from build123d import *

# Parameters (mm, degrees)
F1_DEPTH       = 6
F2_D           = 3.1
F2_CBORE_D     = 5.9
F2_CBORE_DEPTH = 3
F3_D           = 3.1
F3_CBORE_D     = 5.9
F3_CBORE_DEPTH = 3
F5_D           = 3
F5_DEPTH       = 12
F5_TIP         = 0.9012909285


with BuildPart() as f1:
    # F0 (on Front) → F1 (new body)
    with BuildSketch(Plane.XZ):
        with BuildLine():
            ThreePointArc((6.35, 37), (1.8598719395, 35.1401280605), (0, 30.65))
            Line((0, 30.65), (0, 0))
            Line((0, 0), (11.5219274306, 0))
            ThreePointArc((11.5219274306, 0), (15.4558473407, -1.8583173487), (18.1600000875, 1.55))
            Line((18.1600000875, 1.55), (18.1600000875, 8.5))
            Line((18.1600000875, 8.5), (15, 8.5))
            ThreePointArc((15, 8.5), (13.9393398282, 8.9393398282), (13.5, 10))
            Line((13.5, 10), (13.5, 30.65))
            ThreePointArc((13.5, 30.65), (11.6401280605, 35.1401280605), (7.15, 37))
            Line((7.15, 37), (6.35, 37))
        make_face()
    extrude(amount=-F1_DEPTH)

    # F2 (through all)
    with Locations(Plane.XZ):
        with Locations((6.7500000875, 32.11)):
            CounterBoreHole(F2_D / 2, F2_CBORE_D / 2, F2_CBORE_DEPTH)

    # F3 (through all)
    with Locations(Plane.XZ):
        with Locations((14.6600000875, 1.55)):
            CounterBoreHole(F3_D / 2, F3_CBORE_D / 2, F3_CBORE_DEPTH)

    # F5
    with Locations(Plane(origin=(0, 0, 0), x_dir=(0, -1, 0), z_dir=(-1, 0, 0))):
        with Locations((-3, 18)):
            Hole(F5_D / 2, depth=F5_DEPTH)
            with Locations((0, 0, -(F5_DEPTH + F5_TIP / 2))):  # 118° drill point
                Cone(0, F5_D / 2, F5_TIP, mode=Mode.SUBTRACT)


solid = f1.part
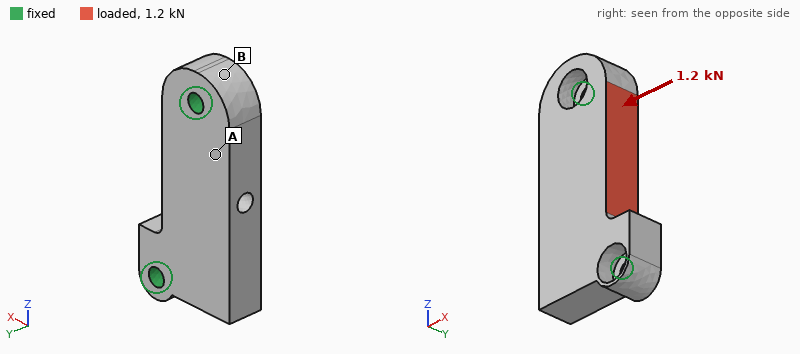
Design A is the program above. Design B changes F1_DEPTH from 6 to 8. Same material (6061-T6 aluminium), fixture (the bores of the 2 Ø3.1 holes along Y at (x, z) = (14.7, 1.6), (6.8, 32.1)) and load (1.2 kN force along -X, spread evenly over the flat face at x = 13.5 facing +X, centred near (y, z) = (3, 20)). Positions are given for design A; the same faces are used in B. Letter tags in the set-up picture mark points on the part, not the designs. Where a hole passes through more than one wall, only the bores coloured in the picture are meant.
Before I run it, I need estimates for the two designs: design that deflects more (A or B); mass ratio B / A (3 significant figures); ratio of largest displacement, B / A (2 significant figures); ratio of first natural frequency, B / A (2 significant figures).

A
1.36
0.53
1.3
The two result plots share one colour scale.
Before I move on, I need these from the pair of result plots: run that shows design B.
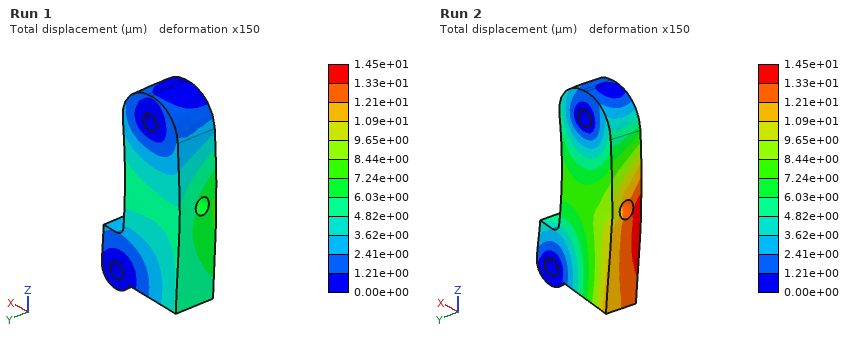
Run 1
